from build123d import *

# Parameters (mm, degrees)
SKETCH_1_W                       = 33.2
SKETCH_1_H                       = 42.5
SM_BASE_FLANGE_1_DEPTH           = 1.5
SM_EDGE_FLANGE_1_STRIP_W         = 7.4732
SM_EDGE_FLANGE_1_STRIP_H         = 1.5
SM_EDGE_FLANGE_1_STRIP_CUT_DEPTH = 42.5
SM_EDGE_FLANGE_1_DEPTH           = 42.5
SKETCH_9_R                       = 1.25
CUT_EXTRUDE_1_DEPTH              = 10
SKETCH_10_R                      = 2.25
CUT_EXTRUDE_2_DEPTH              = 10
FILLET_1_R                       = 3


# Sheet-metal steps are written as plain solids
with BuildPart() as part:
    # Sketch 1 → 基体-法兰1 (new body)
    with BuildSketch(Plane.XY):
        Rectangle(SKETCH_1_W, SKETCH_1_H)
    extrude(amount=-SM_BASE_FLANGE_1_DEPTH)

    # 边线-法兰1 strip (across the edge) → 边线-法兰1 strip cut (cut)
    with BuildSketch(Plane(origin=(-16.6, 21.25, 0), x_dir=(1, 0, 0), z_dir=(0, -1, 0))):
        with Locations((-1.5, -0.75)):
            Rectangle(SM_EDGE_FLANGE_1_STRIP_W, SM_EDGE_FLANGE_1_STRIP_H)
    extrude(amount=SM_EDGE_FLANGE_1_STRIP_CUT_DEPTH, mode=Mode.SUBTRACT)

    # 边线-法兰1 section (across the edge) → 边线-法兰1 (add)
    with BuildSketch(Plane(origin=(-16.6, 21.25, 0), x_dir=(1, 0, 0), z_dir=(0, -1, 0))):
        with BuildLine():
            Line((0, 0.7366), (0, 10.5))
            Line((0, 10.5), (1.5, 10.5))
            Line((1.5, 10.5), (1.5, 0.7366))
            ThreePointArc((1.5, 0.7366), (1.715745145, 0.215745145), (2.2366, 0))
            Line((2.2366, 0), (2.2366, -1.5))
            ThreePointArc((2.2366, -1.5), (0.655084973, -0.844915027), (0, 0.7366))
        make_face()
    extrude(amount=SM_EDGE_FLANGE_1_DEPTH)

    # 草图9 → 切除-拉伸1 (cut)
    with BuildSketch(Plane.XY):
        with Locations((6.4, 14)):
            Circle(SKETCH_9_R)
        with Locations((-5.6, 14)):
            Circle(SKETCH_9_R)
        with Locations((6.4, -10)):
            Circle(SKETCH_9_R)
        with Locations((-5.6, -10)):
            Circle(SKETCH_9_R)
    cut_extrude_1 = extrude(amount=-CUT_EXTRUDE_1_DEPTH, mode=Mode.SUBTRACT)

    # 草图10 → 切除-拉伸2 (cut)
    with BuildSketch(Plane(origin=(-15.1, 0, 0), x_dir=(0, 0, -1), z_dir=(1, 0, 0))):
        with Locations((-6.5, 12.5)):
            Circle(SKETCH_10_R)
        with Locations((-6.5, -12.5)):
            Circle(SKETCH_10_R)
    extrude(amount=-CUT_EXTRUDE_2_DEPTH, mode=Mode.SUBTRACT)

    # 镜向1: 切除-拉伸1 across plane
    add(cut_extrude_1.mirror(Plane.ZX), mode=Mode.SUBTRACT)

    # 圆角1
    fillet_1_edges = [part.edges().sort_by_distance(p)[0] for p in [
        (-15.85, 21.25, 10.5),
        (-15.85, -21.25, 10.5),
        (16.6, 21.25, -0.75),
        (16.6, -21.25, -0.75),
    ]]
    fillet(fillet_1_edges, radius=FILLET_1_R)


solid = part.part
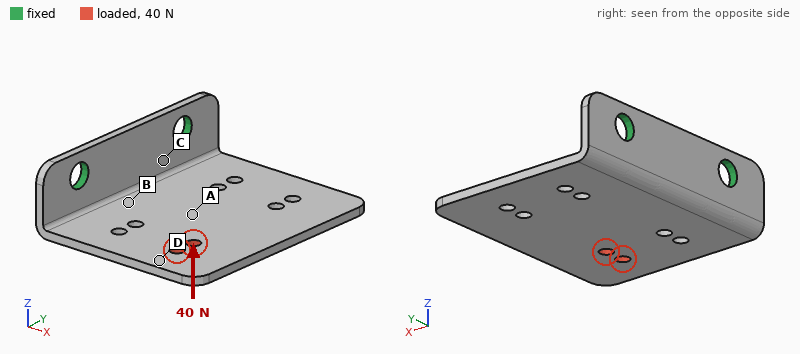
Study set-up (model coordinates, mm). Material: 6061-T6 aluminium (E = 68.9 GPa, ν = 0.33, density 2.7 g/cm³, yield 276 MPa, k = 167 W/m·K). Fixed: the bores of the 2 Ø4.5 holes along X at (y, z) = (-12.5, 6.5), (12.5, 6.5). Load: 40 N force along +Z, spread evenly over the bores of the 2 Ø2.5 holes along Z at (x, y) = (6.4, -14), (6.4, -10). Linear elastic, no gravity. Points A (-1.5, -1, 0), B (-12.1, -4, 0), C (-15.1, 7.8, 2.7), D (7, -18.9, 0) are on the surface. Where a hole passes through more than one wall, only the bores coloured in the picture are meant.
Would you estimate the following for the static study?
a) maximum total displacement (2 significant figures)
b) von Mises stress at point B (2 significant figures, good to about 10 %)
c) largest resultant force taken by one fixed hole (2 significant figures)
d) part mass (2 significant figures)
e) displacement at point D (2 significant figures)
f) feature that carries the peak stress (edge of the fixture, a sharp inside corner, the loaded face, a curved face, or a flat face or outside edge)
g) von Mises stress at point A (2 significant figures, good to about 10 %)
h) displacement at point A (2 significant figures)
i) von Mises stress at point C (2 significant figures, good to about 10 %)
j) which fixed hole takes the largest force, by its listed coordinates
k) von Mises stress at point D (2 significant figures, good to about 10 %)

0.62 mm
50 MPa
37 N
7.1 g
0.41 mm
a flat face or outside edge
29 MPa
0.18 mm
41 MPa
(-12.5, 6.5)
17 MPa
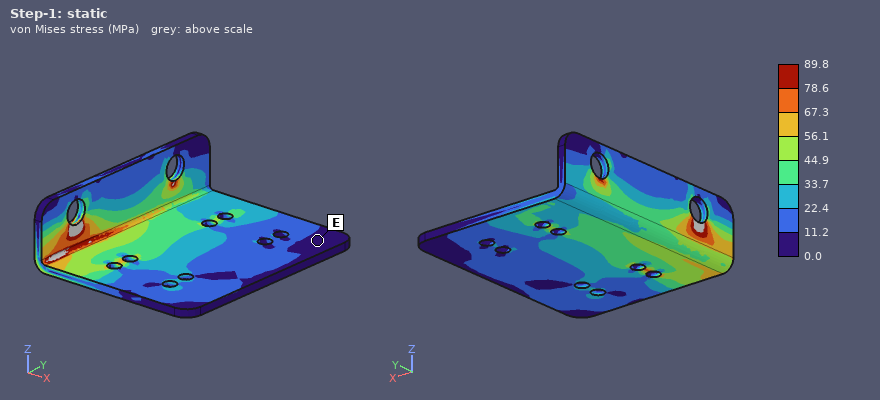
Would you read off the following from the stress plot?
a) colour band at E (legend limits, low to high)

0.0 to 11.2 MPa
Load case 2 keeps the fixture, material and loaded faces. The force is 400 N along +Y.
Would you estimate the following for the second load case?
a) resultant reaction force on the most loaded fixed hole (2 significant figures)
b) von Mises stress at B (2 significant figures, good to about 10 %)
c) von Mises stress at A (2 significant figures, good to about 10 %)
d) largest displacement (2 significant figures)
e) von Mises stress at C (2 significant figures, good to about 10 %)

400 N
62 MPa
32 MPa
0.25 mm
93 MPa
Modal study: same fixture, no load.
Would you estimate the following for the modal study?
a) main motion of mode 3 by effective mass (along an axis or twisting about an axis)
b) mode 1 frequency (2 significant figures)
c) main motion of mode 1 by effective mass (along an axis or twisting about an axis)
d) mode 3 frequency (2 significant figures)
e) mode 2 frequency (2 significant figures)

along Y
910 Hz
along Z
4500 Hz
2100 Hz
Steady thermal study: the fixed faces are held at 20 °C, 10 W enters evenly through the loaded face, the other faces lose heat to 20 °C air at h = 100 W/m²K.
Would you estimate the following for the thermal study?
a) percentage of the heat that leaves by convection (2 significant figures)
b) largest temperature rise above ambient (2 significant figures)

42 %
34 K
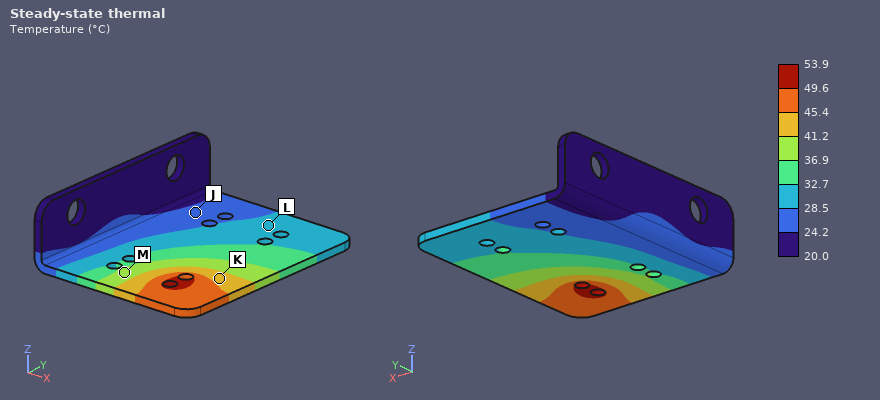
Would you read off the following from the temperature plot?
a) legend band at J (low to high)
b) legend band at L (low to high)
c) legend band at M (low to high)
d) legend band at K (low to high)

24.2 to 28.5 °C
28.5 to 32.7 °C
36.9 to 41.2 °C
41.2 to 45.4 °C
